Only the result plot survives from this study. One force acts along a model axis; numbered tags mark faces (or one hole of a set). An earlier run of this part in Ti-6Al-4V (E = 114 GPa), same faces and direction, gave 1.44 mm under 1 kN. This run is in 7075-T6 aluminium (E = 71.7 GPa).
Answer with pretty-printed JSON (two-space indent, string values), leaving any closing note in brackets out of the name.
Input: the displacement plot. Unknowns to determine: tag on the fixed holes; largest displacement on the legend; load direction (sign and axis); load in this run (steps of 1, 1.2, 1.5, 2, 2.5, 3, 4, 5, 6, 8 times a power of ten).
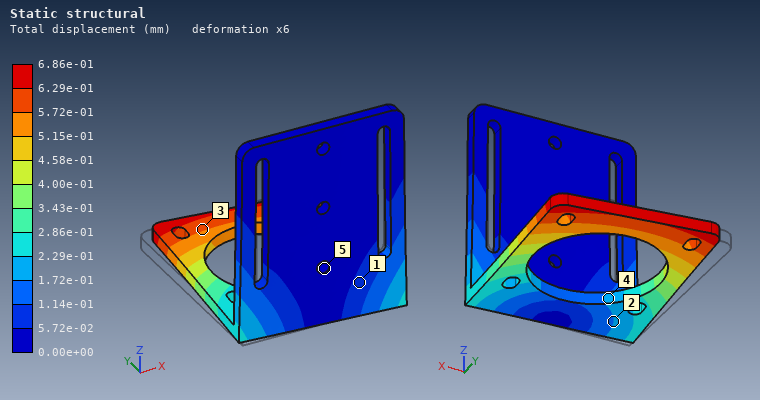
{
  "tag on the fixed holes": "5",
  "largest displacement on the legend": "6.86e-01 mm",
  "load direction": "+X",
  "load in this run": "300 N"
}
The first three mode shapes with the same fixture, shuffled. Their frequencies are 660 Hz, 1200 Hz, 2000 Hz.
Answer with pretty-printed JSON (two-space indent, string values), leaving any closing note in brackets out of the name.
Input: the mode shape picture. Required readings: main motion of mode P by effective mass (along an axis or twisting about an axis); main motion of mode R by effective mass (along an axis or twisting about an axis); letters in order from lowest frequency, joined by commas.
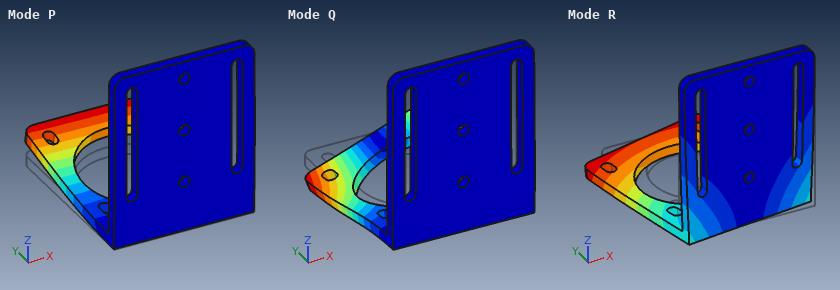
{
  "main motion of mode P by effective mass": "along Z",
  "main motion of mode R by effective mass": "along X",
  "letters in order from lowest frequency, joined by commas": "P, R, Q"
}
